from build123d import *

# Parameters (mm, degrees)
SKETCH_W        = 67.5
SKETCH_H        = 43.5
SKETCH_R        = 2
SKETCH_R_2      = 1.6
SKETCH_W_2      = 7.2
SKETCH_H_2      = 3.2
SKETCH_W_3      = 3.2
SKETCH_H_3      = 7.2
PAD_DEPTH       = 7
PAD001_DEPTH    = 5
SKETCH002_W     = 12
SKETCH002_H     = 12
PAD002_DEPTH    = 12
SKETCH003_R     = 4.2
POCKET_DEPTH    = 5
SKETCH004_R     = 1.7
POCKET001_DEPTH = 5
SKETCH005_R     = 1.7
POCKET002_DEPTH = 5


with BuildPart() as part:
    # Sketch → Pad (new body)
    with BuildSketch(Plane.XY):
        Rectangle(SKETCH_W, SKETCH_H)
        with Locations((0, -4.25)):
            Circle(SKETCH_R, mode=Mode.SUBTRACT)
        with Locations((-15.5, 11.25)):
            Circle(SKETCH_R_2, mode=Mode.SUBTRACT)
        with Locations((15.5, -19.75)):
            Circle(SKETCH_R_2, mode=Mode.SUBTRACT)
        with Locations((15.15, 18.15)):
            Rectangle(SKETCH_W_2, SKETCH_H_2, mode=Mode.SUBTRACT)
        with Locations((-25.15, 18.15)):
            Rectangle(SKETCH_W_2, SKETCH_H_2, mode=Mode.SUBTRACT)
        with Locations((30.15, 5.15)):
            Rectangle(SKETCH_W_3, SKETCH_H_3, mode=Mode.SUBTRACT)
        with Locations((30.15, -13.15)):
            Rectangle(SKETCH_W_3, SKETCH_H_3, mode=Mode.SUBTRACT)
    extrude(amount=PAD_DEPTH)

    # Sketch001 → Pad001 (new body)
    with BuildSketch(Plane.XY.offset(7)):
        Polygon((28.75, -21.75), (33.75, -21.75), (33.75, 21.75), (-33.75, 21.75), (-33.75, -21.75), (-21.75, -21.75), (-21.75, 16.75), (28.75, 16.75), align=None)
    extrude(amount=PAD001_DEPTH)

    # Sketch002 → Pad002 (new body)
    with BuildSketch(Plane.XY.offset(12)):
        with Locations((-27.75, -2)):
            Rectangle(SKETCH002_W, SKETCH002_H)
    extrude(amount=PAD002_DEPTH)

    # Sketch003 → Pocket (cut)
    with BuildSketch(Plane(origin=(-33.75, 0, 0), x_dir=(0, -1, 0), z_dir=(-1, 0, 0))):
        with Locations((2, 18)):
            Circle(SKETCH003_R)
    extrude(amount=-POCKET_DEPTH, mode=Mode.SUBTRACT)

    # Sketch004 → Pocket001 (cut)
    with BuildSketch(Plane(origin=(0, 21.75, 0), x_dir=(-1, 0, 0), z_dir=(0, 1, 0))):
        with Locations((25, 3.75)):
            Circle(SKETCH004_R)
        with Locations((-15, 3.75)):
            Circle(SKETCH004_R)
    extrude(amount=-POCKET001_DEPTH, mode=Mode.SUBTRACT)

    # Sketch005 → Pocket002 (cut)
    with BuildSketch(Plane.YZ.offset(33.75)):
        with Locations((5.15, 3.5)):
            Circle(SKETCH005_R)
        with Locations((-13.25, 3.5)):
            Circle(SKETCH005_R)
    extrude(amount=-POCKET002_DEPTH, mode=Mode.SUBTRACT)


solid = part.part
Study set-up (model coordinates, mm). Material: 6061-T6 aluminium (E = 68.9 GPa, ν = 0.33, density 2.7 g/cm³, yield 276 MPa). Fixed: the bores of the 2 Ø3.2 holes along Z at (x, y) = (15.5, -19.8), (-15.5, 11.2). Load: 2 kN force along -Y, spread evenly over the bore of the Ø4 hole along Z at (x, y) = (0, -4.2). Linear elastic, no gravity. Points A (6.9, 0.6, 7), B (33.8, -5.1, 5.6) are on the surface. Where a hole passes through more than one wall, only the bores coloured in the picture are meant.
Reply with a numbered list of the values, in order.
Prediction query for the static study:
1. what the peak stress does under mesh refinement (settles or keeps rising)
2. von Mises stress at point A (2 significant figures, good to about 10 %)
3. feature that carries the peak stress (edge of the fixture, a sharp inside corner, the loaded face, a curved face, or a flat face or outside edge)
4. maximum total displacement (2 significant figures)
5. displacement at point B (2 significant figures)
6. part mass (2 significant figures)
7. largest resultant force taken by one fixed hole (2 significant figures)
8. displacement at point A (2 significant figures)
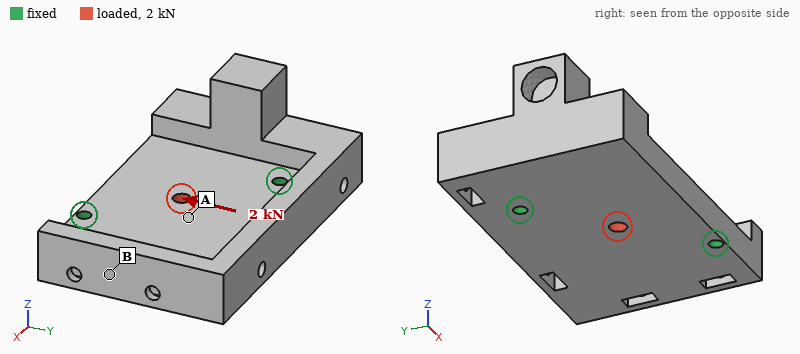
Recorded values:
1. keeps rising
2. 7.8 MPa
3. edge of the fixture
4. 5.4 µm
5. 1.5 µm
6. 70 g
7. 1.0 kN
8. 3.6 µm
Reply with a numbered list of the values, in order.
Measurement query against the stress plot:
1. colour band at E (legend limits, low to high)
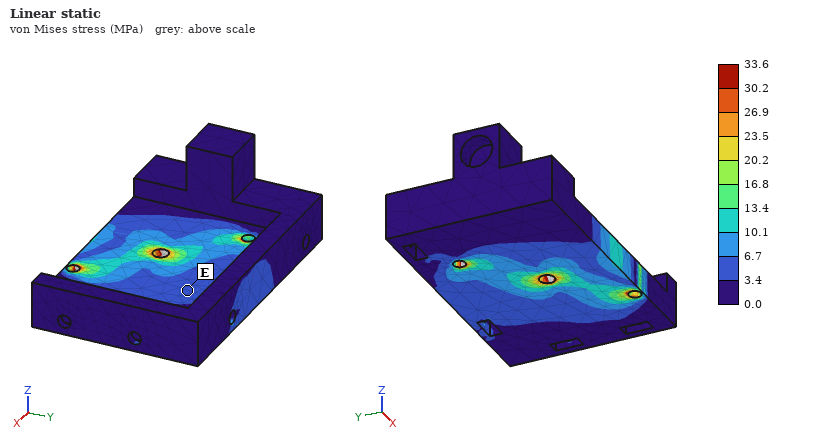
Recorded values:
1. 3.4 to 6.7 MPa
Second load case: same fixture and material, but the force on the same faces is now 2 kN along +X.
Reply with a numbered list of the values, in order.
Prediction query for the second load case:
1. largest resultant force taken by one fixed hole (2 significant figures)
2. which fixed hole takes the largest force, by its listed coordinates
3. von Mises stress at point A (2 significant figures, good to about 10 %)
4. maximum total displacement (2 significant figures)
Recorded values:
1. 1.1 kN
2. (-15.5, 11.2)
3. 8.9 MPa
4. 4.9 µm
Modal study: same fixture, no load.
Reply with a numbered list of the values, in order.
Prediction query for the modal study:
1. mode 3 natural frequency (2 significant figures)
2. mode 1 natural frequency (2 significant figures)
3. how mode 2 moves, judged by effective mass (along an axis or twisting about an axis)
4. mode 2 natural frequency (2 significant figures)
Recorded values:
1. 8800 Hz
2. 3400 Hz
3. along Z
4. 5000 Hz
